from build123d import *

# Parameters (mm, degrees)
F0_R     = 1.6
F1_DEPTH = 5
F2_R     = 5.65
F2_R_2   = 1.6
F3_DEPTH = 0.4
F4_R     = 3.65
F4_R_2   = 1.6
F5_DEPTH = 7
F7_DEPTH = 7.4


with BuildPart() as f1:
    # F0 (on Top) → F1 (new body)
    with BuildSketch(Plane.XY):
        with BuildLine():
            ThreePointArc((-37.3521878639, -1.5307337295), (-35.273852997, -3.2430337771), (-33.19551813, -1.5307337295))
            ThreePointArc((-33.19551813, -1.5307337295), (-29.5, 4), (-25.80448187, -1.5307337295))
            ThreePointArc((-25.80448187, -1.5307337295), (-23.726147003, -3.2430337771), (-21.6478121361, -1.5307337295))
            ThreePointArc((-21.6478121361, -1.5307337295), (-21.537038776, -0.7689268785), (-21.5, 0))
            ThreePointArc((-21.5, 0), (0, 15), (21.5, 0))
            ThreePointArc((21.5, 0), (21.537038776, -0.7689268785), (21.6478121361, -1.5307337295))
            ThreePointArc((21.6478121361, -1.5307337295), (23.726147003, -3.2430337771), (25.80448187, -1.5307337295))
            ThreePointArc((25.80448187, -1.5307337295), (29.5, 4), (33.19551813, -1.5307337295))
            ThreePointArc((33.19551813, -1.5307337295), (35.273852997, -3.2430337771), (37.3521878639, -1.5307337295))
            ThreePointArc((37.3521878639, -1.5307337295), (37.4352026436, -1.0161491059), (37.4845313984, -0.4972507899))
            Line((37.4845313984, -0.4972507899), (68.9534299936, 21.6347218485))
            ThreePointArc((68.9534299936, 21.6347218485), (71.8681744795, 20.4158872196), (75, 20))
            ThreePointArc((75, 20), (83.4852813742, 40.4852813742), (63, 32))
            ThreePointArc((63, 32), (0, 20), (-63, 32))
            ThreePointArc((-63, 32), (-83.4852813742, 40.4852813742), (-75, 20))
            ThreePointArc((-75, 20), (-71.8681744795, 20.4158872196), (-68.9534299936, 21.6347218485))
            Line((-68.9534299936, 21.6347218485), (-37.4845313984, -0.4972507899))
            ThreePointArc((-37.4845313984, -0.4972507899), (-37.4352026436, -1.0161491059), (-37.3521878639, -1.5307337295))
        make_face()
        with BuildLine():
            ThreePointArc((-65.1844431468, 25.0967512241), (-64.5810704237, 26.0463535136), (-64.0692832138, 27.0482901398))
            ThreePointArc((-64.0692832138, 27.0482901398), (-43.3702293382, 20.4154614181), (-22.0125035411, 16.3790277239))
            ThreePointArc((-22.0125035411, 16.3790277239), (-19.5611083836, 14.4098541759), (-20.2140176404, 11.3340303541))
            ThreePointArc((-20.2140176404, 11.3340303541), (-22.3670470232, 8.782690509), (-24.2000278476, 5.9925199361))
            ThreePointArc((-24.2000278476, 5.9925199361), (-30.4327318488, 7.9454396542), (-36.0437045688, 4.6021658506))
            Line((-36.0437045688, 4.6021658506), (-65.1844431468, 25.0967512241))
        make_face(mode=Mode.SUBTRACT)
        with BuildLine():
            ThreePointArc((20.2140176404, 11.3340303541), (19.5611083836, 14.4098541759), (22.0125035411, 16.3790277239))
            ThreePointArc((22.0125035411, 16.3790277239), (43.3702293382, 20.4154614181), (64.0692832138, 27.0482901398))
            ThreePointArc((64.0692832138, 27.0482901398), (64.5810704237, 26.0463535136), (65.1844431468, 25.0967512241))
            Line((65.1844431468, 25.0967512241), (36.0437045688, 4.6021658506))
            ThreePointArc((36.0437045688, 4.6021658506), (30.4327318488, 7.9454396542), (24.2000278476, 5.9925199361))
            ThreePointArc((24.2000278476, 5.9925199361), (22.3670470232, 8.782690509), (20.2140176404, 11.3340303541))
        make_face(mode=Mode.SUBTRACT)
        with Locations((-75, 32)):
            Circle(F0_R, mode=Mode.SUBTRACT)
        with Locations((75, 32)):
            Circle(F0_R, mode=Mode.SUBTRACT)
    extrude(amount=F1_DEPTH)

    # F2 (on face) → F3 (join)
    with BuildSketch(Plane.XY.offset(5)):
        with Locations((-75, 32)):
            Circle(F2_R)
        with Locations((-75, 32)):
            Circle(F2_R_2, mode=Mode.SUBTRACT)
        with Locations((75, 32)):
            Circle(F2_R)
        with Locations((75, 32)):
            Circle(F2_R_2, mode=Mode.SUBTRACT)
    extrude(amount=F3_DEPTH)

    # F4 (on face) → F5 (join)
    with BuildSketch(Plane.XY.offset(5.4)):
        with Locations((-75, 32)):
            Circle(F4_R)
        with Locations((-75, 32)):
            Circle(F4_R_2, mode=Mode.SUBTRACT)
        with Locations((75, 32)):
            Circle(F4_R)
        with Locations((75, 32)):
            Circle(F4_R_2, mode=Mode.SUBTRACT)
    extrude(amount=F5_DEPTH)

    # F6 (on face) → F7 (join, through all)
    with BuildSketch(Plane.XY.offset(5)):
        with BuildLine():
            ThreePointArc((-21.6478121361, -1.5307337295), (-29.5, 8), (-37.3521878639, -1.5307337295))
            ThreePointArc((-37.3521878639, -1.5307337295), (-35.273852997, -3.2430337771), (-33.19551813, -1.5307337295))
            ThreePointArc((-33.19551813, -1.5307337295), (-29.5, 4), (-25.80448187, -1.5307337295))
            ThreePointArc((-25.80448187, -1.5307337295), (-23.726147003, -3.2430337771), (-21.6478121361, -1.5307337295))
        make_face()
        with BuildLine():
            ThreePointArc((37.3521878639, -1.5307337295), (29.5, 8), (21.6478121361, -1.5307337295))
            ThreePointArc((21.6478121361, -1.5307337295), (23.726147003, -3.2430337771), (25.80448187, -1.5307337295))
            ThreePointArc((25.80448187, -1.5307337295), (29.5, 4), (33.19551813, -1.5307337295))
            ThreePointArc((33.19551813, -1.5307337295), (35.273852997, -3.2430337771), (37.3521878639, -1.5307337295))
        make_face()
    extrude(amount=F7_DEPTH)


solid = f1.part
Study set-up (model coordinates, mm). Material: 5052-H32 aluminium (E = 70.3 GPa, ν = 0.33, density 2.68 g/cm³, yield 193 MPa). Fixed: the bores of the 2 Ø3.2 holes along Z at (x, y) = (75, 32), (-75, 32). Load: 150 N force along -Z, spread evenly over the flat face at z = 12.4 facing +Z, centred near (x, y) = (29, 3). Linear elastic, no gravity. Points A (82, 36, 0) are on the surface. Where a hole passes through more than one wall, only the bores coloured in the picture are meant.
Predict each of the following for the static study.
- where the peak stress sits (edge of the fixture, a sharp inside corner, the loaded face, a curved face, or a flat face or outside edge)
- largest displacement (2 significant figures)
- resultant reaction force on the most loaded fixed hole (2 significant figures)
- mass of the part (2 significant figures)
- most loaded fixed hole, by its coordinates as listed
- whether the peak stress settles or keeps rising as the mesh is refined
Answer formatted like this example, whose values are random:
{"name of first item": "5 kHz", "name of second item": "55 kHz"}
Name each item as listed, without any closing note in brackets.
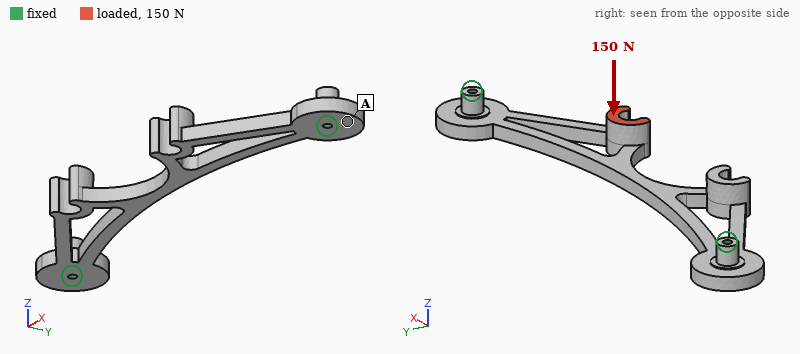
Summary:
{"where the peak stress sits": "edge of the fixture", "largest displacement": "0.55 mm", "resultant reaction force on the most loaded fixed hole": "120 N", "mass of the part": "36 g", "most loaded fixed hole, by its coordinates as listed": "(75, 32)", "whether the peak stress settles or keeps rising as the mesh is refined": "keeps rising"}
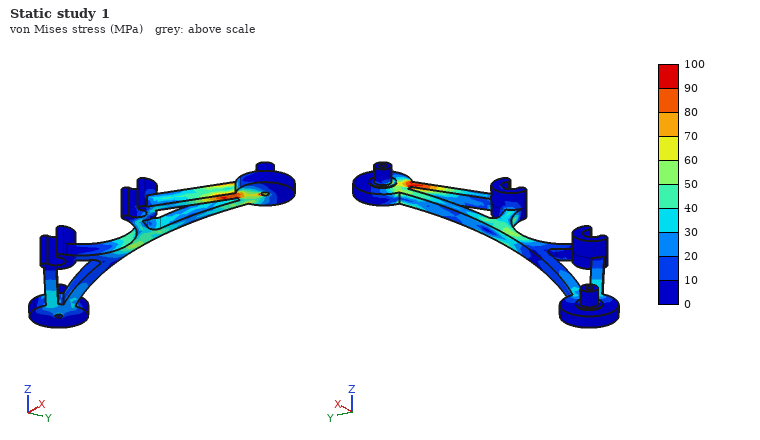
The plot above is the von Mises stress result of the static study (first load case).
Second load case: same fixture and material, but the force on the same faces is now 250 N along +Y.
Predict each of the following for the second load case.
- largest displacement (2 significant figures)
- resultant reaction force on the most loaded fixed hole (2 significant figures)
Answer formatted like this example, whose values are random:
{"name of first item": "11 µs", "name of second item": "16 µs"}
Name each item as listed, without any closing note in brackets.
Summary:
{"largest displacement": "0.41 mm", "resultant reaction force on the most loaded fixed hole": "380 N"}
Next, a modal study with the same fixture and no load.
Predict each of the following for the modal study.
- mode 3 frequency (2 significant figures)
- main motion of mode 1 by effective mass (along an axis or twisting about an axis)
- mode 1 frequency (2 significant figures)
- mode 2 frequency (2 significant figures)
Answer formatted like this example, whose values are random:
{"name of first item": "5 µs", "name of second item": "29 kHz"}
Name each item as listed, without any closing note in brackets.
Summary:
{"mode 3 frequency": "2300 Hz", "main motion of mode 1 by effective mass": "along Z", "mode 1 frequency": "920 Hz", "mode 2 frequency": "1900 Hz"}
